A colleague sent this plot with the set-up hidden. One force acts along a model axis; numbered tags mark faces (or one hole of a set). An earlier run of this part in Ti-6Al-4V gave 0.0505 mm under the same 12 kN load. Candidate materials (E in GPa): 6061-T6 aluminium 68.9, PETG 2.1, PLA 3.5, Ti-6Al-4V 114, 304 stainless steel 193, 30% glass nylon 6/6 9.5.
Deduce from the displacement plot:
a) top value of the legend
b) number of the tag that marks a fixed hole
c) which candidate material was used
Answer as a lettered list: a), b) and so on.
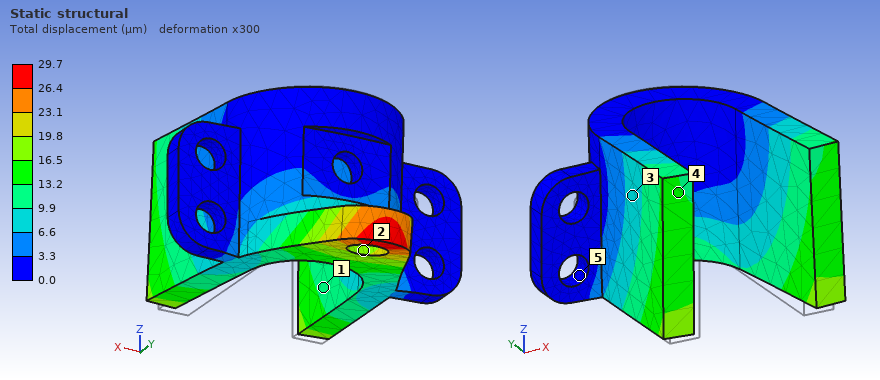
a) 29.7 µm
b) 5
c) 304 stainless steel
